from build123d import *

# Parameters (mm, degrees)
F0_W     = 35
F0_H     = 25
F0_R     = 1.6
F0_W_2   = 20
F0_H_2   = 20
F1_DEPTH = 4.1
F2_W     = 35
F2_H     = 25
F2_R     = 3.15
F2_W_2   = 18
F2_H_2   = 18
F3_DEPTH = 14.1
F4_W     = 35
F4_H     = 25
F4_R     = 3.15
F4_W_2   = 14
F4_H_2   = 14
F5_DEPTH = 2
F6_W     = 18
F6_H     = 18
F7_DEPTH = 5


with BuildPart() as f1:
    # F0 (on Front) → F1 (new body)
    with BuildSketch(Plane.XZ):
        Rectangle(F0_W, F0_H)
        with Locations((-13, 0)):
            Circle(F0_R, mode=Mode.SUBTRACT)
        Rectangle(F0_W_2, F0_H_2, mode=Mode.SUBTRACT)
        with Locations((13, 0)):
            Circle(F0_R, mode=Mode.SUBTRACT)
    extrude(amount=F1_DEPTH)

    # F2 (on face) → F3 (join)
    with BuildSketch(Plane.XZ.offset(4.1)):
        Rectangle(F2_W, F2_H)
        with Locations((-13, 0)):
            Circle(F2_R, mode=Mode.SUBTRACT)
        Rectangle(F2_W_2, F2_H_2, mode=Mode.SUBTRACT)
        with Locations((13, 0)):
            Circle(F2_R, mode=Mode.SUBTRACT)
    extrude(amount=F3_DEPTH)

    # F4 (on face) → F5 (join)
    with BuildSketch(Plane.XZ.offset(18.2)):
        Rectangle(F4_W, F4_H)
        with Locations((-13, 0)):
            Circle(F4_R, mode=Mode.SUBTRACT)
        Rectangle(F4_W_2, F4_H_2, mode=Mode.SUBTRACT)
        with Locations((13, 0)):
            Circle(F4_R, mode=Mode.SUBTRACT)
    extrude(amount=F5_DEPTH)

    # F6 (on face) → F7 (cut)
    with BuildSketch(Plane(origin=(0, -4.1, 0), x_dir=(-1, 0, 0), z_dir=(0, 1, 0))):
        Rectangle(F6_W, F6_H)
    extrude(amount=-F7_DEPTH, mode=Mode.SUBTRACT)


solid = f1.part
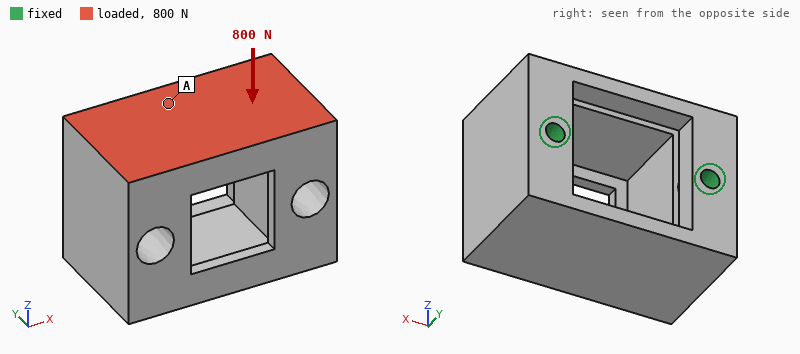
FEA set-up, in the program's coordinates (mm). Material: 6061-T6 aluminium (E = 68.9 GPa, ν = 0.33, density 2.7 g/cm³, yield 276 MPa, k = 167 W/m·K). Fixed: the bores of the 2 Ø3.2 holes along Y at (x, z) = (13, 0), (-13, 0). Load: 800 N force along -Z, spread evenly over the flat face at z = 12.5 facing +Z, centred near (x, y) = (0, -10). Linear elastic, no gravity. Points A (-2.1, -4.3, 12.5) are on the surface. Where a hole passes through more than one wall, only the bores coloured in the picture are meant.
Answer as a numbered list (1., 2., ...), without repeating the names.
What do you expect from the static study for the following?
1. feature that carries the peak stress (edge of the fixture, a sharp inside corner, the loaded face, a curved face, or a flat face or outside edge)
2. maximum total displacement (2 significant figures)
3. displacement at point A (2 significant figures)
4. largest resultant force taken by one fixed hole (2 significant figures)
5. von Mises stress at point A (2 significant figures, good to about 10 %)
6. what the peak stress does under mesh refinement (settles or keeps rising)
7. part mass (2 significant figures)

1. edge of the fixture
2. 28 µm
3. 16 µm
4. 400 N
5. 14 MPa
6. keeps rising
7. 27 g
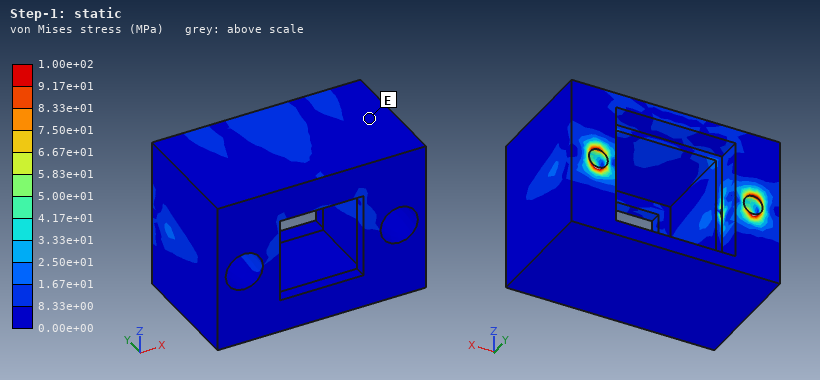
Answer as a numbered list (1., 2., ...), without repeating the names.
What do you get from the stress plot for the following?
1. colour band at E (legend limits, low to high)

1. 0.00e+00 to 8.33e+00 MPa
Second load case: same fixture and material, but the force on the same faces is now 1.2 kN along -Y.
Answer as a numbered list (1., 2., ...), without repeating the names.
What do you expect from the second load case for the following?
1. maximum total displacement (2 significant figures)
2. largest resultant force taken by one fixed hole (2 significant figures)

1. 61 µm
2. 600 N
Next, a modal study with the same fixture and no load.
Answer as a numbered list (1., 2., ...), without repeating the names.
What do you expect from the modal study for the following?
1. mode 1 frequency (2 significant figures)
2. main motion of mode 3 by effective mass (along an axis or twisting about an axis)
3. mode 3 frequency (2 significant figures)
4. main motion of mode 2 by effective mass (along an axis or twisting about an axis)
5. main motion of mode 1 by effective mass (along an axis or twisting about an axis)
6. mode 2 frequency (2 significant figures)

1. 5500 Hz
2. along X
3. 13 kHz
4. twisting about Y
5. along Z
6. 12 kHz
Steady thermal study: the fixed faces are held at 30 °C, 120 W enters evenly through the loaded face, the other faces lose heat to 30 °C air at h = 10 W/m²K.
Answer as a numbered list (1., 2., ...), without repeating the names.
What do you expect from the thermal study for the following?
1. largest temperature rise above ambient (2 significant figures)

1. 70 K
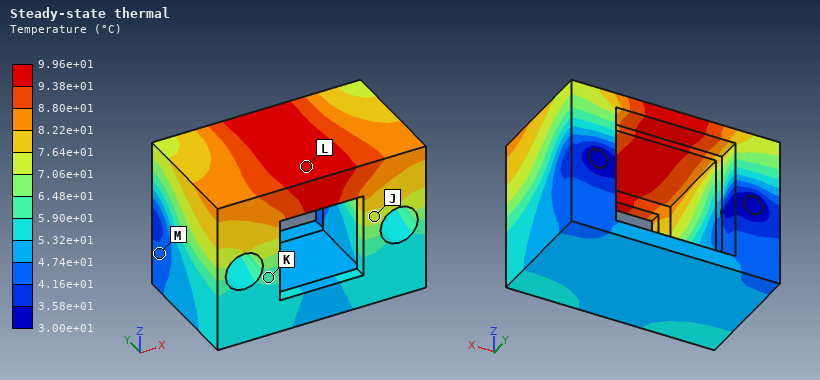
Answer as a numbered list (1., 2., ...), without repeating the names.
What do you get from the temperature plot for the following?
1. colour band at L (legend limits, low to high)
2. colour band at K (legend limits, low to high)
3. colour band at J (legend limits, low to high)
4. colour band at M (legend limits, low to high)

1. 9.38e+01 to 9.96e+01 °C
2. 5.90e+01 to 6.48e+01 °C
3. 7.06e+01 to 7.64e+01 °C
4. 4.16e+01 to 4.74e+01 °C
